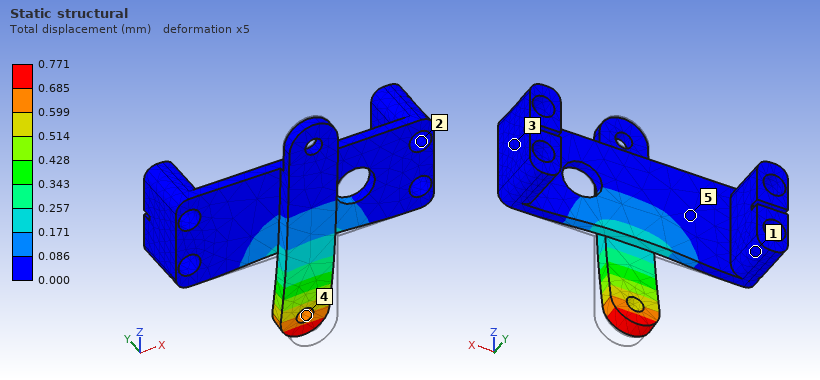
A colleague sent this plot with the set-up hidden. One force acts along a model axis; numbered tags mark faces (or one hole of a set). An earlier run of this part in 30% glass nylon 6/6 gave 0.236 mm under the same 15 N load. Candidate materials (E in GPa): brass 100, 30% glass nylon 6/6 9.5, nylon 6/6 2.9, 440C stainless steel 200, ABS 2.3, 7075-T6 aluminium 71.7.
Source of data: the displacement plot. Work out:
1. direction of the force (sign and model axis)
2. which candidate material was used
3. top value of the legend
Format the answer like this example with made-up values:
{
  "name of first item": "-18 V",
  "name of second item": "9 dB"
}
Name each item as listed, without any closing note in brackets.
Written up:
{
  "direction of the force": "+Y",
  "which candidate material was used": "nylon 6/6",
  "top value of the legend": "0.771 mm"
}
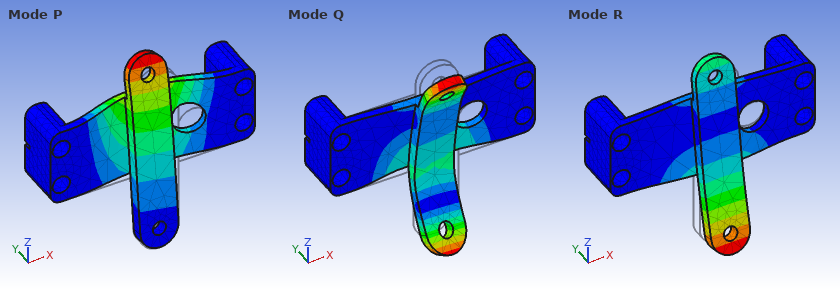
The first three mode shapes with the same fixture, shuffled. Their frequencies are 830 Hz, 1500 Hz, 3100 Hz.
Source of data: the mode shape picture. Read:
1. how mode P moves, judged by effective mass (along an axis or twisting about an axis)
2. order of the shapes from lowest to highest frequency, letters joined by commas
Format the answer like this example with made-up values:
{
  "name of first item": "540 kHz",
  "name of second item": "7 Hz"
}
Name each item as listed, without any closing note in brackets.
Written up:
{
  "how mode P moves, judged by effective mass": "along Y",
  "order of the shapes from lowest to highest frequency, letters joined by commas": "R, P, Q"
}
